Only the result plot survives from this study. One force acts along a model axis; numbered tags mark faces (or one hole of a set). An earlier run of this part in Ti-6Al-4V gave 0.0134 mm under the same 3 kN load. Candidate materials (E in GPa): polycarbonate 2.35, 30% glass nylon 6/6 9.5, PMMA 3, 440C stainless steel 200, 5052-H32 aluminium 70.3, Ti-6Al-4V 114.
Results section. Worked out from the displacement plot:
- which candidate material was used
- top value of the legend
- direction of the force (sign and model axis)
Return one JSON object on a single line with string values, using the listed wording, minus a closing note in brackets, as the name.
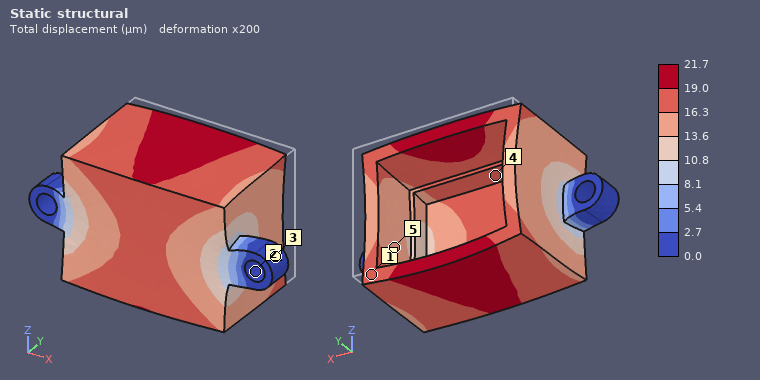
{"which candidate material was used": "5052-H32 aluminium", "top value of the legend": "21.7 µm", "direction of the force": "-Y"}
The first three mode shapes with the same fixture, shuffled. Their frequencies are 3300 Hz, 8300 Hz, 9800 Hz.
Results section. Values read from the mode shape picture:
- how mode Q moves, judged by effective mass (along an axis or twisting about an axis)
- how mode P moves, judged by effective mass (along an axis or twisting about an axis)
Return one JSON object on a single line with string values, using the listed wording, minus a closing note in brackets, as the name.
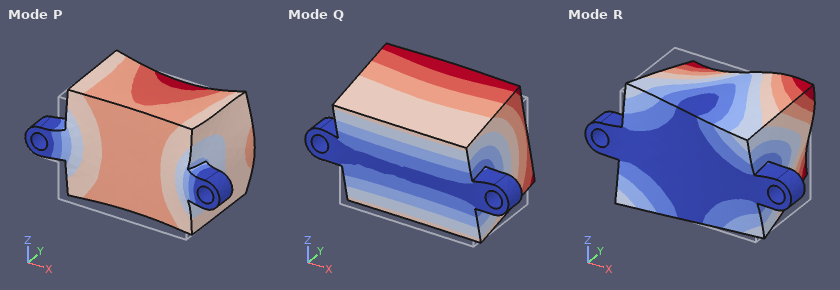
{"how mode Q moves, judged by effective mass": "along Z", "how mode P moves, judged by effective mass": "along Y"}
